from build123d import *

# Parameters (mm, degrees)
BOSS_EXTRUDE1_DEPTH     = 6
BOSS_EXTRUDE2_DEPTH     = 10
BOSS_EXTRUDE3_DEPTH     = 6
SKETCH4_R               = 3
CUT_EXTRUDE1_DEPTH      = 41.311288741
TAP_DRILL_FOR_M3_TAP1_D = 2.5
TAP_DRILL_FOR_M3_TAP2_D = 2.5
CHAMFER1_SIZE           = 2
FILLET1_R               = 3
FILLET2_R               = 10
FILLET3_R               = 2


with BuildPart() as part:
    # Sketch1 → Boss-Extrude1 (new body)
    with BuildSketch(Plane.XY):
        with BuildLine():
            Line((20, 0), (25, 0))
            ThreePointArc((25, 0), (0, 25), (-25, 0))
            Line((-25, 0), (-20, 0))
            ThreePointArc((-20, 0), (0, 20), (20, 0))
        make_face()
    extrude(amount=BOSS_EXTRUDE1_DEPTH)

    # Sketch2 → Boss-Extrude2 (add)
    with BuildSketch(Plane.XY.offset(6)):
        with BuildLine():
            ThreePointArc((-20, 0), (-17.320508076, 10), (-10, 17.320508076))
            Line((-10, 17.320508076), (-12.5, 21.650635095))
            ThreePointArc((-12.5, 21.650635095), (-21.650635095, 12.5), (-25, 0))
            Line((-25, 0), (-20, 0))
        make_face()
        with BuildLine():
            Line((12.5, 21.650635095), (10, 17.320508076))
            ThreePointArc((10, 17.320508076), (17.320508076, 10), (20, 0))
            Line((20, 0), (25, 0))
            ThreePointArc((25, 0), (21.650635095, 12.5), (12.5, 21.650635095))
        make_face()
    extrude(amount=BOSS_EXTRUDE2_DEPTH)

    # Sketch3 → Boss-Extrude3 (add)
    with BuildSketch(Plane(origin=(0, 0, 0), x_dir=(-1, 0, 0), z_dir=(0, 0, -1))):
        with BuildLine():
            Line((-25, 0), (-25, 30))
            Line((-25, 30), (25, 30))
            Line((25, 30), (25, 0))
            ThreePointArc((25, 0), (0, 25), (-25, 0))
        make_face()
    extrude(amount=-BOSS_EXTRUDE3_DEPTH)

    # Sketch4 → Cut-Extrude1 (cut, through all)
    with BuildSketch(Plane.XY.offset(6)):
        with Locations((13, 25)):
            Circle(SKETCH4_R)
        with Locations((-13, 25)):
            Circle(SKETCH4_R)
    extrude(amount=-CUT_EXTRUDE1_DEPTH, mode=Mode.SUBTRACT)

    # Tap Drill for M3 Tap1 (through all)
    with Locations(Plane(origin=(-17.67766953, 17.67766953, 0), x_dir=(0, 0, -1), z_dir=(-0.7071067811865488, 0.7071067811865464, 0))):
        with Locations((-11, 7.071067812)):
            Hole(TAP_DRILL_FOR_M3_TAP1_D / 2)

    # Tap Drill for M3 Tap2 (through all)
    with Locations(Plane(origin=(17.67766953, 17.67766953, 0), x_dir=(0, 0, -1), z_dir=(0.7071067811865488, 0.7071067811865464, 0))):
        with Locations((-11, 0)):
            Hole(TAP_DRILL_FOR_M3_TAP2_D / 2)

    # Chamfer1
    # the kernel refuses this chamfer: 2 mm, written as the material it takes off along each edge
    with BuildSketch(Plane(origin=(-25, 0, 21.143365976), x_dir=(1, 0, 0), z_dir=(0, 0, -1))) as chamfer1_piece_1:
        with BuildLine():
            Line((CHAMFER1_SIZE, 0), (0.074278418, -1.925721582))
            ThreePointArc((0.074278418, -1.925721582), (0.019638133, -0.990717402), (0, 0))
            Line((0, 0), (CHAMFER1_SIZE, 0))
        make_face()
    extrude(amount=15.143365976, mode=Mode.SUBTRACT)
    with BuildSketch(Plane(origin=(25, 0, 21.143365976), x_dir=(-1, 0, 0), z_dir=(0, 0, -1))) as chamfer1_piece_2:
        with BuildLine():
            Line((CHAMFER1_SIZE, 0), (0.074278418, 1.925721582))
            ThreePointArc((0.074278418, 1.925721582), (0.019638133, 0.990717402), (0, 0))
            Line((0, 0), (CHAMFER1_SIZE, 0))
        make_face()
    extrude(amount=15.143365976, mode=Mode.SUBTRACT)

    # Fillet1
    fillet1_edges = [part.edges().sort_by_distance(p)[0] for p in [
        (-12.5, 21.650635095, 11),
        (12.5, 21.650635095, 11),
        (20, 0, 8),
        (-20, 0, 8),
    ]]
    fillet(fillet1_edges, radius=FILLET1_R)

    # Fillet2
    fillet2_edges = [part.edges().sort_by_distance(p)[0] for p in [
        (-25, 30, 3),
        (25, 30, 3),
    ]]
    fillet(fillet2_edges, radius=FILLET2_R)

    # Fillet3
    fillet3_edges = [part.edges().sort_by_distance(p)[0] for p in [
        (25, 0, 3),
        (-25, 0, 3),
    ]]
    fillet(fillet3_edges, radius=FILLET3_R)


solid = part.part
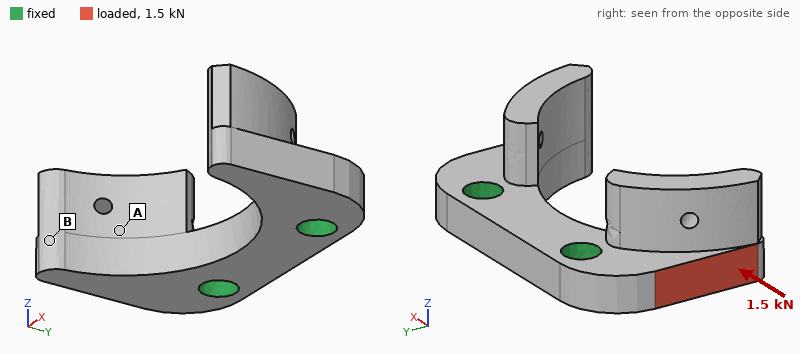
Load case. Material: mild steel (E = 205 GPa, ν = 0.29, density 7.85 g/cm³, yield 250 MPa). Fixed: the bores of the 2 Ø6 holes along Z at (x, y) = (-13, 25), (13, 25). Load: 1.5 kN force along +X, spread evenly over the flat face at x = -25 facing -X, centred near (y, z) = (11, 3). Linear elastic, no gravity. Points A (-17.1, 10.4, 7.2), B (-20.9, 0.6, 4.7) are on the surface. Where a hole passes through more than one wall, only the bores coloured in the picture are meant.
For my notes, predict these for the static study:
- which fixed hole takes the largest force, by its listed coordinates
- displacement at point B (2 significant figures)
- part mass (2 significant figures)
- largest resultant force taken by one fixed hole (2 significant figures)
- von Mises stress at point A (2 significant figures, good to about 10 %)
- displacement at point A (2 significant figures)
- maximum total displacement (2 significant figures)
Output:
(-13, 25)
23 µm
53 g
1.3 kN
36 MPa
10.0 µm
26 µm
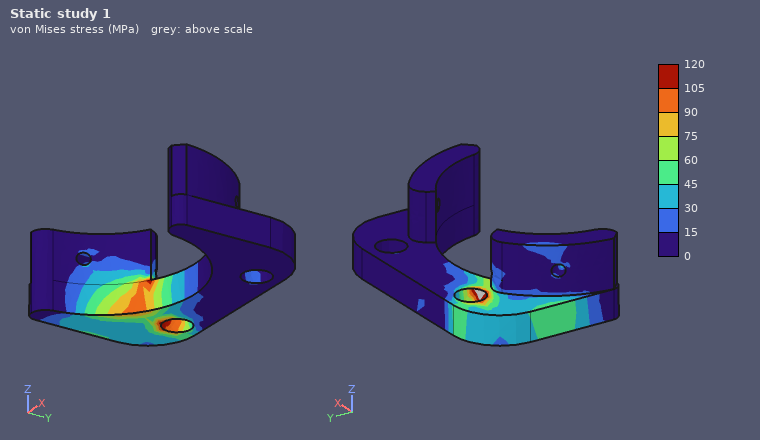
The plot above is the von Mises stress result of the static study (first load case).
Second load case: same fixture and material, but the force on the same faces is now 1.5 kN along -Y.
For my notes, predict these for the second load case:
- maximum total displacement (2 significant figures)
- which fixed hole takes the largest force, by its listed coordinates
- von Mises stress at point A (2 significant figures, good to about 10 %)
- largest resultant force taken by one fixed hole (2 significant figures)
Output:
23 µm
(-13, 25)
23 MPa
1.7 kN
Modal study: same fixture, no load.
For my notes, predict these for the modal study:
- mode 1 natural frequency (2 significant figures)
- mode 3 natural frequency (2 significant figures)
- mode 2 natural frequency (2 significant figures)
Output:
7300 Hz
11 kHz
7400 Hz
